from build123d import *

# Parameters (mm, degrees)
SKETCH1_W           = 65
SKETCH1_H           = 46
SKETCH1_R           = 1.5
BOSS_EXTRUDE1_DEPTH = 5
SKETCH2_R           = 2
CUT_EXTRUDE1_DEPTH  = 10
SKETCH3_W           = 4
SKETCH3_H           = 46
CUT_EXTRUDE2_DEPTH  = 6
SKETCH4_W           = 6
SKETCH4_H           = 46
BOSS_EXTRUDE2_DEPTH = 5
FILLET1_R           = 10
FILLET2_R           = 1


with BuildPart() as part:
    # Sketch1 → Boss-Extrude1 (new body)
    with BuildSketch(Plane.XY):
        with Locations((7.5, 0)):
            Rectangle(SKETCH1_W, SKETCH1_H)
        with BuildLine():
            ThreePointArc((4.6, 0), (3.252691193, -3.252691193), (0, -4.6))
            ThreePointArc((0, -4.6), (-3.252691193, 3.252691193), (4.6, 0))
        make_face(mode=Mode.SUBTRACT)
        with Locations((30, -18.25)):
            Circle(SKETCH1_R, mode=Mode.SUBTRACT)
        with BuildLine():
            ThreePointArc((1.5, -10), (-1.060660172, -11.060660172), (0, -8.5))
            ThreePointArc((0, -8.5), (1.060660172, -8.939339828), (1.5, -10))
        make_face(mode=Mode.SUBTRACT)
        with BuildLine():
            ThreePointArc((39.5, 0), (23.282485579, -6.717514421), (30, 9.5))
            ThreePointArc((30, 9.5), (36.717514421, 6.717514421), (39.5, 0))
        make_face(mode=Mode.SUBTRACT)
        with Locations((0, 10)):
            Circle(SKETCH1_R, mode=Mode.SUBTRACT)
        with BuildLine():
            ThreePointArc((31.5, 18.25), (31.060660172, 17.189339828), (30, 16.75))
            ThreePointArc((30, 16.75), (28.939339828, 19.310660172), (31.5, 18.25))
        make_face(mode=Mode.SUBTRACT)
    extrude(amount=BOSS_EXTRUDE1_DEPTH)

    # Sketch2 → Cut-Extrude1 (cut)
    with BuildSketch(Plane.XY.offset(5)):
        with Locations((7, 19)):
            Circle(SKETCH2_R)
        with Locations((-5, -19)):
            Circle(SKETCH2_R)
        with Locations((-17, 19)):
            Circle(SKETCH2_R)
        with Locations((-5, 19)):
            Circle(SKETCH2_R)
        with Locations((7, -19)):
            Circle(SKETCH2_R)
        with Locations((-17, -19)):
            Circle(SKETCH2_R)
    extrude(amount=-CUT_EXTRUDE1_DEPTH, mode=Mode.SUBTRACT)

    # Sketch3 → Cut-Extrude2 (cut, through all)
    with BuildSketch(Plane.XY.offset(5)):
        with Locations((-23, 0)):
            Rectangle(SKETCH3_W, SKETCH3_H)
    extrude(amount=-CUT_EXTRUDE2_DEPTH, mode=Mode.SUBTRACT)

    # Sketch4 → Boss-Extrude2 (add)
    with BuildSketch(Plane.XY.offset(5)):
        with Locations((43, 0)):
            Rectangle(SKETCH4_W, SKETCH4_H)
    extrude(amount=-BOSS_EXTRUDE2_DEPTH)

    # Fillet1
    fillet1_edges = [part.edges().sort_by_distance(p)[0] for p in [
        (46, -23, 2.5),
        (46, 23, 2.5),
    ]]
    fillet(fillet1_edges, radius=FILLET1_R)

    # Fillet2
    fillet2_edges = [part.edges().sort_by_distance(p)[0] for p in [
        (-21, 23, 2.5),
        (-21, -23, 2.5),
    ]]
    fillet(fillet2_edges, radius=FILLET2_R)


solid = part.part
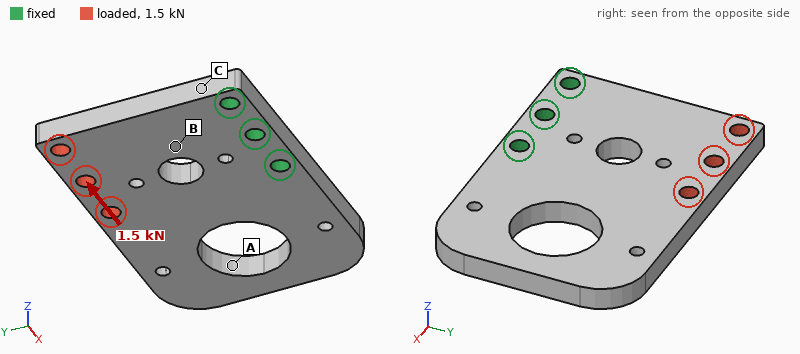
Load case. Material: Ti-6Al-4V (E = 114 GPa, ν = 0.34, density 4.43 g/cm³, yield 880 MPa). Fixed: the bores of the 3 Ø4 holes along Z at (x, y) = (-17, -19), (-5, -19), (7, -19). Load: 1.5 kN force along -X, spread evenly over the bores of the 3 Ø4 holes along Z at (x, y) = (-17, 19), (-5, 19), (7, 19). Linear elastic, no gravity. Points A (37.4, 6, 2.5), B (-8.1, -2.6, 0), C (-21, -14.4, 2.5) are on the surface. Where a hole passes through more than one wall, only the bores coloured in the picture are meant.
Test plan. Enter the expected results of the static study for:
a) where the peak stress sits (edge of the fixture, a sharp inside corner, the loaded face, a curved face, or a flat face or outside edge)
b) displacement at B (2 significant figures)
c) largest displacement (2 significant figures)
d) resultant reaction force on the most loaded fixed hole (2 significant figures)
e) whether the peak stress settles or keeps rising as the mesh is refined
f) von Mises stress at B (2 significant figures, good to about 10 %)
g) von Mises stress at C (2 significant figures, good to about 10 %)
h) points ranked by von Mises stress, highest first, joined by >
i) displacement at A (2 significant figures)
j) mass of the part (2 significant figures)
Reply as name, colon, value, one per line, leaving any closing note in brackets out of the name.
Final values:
where the peak stress sits: edge of the fixture
displacement at B: 8.0 µm
largest displacement: 37 µm
resultant reaction force on the most loaded fixed hole: 2.1 kN
whether the peak stress settles or keeps rising as the mesh is refined: keeps rising
von Mises stress at B: 27 MPa
von Mises stress at C: 50 MPa
points ranked by von Mises stress, highest first, joined by >: C > B > A
displacement at A: 28 µm
mass of the part: 57 g
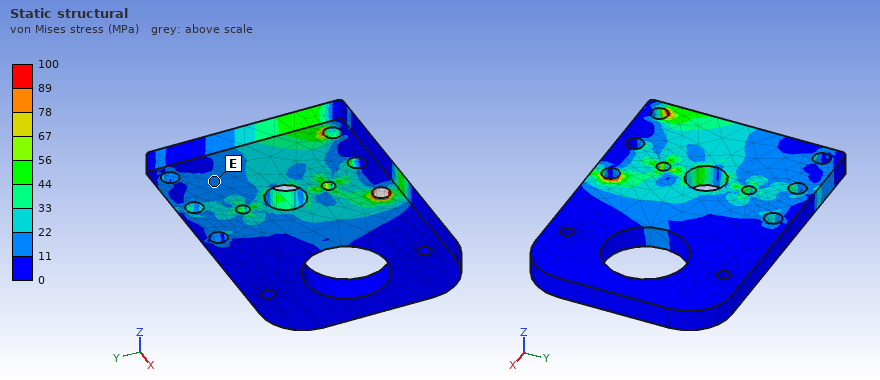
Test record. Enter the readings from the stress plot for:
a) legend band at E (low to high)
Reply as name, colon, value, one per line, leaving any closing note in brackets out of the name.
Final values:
legend band at E: 11 to 22 MPa
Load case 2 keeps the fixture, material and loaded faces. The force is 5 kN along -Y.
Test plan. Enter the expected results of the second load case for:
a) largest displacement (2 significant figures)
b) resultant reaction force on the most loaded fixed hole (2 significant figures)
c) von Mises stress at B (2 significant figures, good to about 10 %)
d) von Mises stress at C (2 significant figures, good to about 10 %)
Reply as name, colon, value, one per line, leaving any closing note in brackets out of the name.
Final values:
largest displacement: 15 µm
resultant reaction force on the most loaded fixed hole: 1.9 kN
von Mises stress at B: 39 MPa
von Mises stress at C: 32 MPa
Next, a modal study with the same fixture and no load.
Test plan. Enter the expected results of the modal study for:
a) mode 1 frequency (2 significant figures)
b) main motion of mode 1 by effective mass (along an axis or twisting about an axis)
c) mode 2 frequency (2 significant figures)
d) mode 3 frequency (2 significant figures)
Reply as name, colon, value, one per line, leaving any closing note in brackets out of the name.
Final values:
mode 1 frequency: 1600 Hz
main motion of mode 1 by effective mass: along Z
mode 2 frequency: 2600 Hz
mode 3 frequency: 4800 Hz
